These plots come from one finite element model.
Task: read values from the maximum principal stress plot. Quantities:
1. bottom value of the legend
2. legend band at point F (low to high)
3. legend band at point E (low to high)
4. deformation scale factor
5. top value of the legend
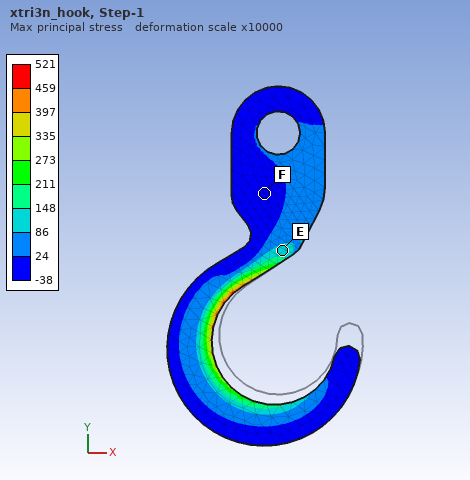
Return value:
-38
-38 to 24
86 to 148
10000
521
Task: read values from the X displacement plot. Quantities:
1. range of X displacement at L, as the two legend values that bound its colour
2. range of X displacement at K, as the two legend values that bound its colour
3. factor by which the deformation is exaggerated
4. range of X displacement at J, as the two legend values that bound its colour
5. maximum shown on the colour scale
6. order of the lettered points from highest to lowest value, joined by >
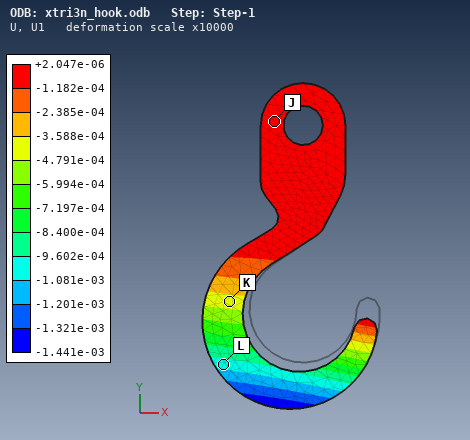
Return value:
-1.081e-03 to -9.602e-04
-4.791e-04 to -3.588e-04
10000
-1.182e-04 to +2.047e-06
+2.047e-06
J > K > L
